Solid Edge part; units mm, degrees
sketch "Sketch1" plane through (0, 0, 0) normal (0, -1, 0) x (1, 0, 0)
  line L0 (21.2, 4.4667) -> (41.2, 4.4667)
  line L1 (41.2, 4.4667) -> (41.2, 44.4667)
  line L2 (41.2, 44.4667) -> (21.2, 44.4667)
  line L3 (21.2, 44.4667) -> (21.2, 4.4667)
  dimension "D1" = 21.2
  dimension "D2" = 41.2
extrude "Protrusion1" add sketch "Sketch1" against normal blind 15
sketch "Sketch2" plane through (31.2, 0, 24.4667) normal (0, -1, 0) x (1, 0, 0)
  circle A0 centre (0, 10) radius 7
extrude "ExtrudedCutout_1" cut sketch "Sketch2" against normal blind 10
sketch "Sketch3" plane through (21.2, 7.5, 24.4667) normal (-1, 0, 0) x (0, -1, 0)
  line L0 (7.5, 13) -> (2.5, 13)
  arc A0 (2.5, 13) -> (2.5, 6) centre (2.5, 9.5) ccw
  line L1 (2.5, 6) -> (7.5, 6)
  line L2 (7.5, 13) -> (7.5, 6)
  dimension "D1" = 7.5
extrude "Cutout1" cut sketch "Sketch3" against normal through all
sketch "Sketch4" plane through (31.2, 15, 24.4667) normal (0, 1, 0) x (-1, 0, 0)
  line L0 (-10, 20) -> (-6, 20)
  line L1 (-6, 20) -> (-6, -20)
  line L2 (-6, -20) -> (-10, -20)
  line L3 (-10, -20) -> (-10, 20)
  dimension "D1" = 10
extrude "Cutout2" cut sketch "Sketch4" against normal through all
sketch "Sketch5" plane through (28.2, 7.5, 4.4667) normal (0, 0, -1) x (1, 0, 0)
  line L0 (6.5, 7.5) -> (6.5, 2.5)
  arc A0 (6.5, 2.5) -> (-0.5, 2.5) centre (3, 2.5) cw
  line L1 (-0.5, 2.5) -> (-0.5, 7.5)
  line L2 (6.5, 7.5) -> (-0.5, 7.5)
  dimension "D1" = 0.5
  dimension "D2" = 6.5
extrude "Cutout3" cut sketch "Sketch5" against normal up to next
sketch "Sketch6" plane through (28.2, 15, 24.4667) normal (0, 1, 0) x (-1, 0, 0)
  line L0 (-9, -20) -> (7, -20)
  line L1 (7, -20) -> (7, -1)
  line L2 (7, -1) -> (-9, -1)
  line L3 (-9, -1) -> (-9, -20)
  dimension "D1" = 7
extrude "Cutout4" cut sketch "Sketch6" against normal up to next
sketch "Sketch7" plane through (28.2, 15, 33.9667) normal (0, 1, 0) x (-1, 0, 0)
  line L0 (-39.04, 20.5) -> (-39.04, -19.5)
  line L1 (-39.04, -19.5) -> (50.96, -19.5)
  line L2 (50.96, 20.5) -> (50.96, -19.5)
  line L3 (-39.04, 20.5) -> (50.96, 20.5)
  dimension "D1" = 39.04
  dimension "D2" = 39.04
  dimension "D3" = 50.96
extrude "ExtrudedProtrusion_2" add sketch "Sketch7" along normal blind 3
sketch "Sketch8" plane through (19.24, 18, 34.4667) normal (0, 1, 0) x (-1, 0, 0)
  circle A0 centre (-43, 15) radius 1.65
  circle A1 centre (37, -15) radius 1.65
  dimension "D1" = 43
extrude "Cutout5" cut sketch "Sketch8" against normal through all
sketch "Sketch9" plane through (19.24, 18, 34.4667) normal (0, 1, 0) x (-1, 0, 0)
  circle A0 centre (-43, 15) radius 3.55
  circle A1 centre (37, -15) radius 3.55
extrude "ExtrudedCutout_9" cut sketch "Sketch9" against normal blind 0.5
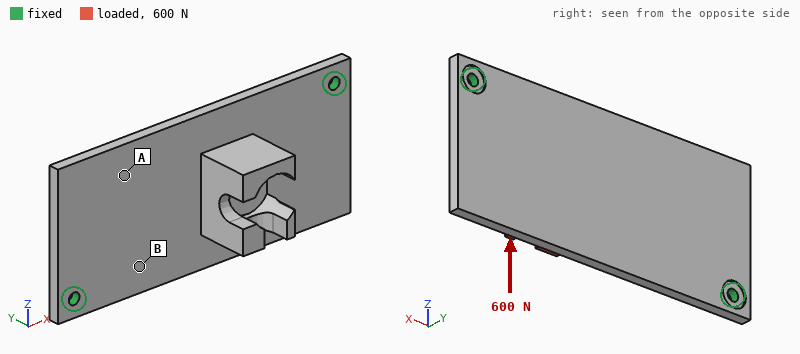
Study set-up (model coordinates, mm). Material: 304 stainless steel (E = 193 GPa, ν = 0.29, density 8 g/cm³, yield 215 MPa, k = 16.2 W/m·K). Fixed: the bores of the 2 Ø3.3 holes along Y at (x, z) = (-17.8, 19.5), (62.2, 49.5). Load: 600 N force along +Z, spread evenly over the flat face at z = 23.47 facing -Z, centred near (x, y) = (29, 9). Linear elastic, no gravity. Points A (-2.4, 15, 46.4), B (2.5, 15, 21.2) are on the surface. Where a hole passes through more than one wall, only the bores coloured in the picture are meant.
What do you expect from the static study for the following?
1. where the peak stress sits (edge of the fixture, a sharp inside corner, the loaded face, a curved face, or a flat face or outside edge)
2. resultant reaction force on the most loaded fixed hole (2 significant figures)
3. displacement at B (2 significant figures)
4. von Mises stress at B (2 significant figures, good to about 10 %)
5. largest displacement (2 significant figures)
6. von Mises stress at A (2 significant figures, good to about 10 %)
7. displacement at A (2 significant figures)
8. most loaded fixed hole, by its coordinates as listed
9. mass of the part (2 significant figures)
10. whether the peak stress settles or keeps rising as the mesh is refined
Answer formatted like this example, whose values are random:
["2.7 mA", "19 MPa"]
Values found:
["edge of the fixture", "350 N", "0.024 mm", "44 MPa", "0.11 mm", "17 MPa", "0.060 mm", "(62.2, 49.5)", "110 g", "keeps rising"]
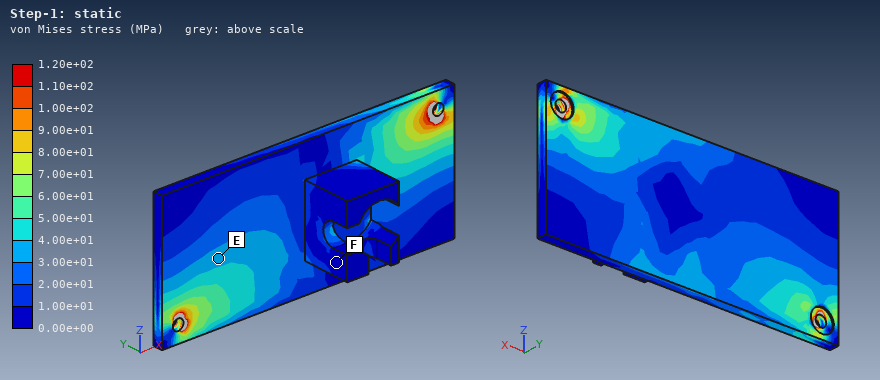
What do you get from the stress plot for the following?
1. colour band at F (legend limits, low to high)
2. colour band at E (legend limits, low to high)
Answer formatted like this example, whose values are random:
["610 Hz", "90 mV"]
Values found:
["0.00e+00 to 1.00e+01 MPa", "3.00e+01 to 4.00e+01 MPa"]
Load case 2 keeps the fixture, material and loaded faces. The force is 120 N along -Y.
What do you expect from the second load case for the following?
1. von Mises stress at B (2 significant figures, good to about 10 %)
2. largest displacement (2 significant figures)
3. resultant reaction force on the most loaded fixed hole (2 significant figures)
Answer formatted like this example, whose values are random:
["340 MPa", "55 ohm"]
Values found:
["17 MPa", "58 µm", "63 N"]
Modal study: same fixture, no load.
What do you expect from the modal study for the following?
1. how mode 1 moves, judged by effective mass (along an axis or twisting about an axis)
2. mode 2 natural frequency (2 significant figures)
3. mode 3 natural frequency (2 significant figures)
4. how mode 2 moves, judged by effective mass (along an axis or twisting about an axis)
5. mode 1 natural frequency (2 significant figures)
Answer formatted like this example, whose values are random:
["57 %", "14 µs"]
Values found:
["along Y", "1400 Hz", "3200 Hz", "along Y", "1300 Hz"]
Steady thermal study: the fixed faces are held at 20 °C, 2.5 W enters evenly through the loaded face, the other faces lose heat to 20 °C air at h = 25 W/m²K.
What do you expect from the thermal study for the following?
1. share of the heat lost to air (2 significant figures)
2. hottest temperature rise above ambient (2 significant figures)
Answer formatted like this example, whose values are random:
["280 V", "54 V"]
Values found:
["75 %", "26 K"]
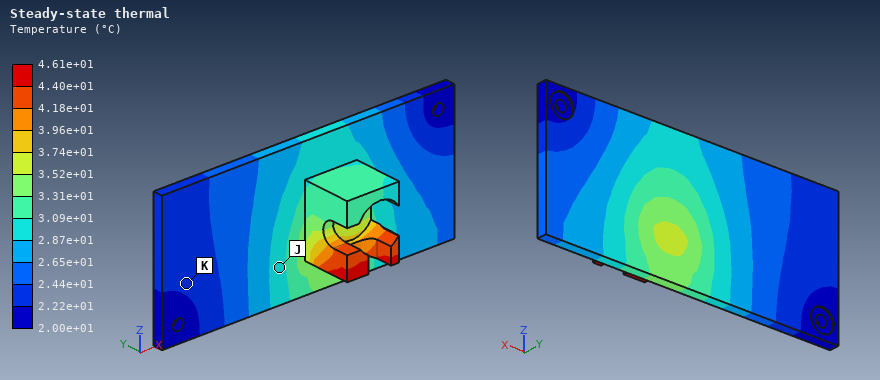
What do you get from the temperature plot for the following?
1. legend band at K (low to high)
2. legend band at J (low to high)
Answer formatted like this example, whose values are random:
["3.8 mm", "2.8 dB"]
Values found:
["2.22e+01 to 2.44e+01 °C", "2.87e+01 to 3.09e+01 °C"]
